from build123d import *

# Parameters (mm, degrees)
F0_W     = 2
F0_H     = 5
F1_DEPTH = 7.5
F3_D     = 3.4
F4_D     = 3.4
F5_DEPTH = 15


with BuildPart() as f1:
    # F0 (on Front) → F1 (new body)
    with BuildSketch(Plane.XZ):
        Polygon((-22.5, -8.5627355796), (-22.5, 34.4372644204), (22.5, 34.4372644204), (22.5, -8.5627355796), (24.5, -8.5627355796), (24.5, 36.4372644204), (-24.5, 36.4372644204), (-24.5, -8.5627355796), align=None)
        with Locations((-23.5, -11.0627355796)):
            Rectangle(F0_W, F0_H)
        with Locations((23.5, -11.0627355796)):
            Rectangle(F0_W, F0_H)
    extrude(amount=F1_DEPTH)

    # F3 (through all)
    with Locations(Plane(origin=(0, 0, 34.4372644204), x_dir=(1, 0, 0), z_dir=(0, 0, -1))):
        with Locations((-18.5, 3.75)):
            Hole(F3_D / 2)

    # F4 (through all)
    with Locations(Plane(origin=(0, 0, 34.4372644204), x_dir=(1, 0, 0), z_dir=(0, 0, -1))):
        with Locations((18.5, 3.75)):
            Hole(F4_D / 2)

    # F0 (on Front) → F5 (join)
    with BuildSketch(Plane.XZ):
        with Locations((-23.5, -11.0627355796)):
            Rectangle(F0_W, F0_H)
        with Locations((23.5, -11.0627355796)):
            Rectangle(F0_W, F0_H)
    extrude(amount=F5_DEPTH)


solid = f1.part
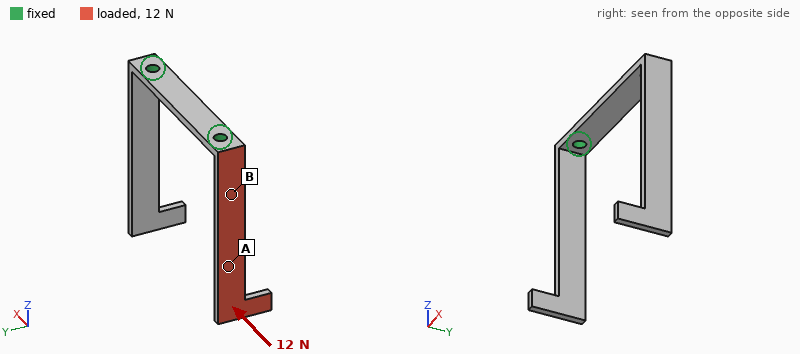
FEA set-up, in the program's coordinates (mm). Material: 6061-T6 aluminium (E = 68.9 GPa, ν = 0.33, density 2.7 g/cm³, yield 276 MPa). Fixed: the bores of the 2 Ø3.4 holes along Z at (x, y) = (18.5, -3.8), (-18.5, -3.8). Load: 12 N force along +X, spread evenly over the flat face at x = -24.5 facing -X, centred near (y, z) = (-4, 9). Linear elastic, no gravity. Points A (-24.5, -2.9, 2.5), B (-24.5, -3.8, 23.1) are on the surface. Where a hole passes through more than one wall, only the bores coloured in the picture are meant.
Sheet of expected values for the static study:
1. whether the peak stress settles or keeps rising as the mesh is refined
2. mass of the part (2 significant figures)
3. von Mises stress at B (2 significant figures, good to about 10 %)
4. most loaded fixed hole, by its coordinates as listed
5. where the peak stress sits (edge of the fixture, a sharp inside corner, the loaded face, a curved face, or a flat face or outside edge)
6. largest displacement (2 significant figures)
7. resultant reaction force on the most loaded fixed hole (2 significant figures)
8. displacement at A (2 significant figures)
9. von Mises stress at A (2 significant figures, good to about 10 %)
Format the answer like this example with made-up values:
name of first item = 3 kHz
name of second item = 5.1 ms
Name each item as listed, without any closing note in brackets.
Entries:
whether the peak stress settles or keeps rising as the mesh is refined = keeps rising
mass of the part = 6.2 g
von Mises stress at B = 37 MPa
most loaded fixed hole, by its coordinates as listed = (-18.5, -3.8)
where the peak stress sits = edge of the fixture
largest displacement = 0.71 mm
resultant reaction force on the most loaded fixed hole = 12 N
displacement at A = 0.41 mm
von Mises stress at A = 8.8 MPa
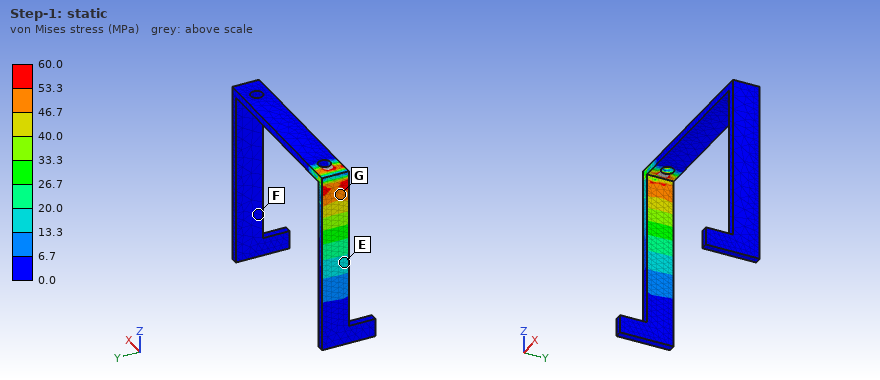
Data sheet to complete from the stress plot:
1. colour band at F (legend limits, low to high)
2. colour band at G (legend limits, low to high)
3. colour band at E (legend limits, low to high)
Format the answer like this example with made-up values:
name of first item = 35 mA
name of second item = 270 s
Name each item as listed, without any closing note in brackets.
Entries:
colour band at F = 0.0 to 6.7 MPa
colour band at G = 46.7 to 53.3 MPa
colour band at E = 13.3 to 20.0 MPa
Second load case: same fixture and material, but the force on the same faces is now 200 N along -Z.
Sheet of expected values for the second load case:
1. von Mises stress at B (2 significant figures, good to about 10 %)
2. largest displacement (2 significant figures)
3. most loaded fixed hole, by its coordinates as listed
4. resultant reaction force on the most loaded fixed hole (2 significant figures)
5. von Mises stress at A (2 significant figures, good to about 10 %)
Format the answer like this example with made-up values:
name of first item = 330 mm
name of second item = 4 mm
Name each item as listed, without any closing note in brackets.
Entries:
von Mises stress at B = 40 MPa
largest displacement = 0.79 mm
most loaded fixed hole, by its coordinates as listed = (-18.5, -3.8)
resultant reaction force on the most loaded fixed hole = 200 N
von Mises stress at A = 19 MPa
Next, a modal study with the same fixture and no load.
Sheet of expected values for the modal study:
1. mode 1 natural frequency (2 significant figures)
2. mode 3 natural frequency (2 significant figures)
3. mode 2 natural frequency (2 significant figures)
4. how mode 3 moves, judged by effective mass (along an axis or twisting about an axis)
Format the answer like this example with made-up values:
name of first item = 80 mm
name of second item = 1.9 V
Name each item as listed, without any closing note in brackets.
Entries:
mode 1 natural frequency = 530 Hz
mode 3 natural frequency = 1200 Hz
mode 2 natural frequency = 530 Hz
how mode 3 moves, judged by effective mass = along Y
